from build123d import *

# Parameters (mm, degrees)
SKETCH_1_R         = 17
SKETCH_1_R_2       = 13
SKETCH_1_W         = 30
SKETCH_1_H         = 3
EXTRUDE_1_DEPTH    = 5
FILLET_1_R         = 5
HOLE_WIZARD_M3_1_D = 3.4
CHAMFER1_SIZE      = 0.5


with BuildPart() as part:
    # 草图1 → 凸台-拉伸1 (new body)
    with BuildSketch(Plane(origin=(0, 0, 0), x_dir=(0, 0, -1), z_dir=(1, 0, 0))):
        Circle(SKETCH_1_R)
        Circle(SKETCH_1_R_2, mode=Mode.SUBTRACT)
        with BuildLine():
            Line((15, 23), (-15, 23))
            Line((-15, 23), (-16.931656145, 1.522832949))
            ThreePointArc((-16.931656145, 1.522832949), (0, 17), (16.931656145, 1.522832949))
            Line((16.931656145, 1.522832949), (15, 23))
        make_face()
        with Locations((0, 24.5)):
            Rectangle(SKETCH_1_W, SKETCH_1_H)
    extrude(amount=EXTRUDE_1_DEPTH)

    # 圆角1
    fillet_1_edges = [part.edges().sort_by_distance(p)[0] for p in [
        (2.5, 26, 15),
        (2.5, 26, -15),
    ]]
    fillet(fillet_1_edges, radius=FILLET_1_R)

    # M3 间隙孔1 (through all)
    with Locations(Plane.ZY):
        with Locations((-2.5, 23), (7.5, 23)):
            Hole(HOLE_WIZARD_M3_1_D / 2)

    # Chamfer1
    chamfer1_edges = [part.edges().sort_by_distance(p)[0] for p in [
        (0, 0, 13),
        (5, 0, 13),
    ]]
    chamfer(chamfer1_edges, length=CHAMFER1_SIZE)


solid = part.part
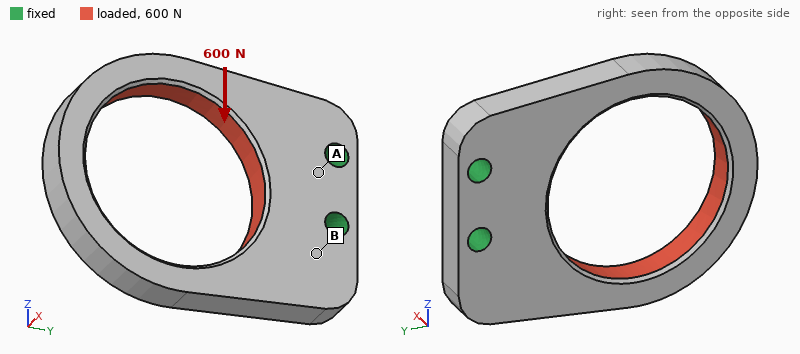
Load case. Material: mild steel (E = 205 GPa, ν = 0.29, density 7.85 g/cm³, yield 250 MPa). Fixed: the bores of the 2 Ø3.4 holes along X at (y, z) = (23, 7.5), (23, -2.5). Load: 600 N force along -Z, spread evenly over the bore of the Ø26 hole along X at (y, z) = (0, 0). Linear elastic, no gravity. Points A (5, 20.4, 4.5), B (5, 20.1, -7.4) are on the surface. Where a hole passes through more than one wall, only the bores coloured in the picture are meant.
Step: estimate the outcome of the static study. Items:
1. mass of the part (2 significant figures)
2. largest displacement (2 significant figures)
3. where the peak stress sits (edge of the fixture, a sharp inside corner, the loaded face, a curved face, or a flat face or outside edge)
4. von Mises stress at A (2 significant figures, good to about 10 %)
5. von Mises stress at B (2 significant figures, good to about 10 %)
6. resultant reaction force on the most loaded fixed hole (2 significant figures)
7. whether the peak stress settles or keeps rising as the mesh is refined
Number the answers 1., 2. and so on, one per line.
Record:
1. 28 g
2. 35 µm
3. edge of the fixture
4. 30 MPa
5. 14 MPa
6. 980 N
7. keeps rising
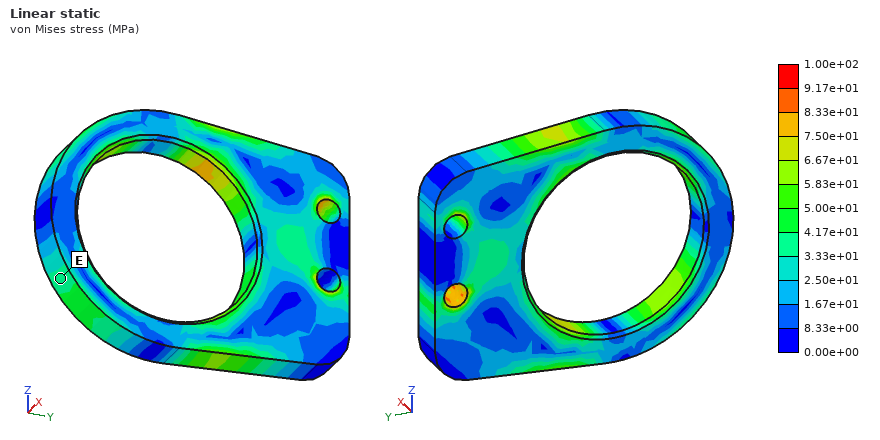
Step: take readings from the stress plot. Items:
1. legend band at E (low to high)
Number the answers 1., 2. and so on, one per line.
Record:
1. 3.33e+01 to 4.17e+01 MPa
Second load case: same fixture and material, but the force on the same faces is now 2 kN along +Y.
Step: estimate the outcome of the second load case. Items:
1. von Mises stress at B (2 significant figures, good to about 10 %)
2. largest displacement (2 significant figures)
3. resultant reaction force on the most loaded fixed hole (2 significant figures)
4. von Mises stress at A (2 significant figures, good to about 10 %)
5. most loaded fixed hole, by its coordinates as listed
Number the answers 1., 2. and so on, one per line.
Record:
1. 40 MPa
2. 21 µm
3. 1.5 kN
4. 15 MPa
5. (23, -2.5)
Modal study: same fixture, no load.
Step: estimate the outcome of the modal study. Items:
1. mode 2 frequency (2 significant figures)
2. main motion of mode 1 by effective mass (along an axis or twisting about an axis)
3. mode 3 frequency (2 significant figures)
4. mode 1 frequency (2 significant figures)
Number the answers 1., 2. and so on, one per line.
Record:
1. 5900 Hz
2. along X
3. 6200 Hz
4. 2900 Hz
